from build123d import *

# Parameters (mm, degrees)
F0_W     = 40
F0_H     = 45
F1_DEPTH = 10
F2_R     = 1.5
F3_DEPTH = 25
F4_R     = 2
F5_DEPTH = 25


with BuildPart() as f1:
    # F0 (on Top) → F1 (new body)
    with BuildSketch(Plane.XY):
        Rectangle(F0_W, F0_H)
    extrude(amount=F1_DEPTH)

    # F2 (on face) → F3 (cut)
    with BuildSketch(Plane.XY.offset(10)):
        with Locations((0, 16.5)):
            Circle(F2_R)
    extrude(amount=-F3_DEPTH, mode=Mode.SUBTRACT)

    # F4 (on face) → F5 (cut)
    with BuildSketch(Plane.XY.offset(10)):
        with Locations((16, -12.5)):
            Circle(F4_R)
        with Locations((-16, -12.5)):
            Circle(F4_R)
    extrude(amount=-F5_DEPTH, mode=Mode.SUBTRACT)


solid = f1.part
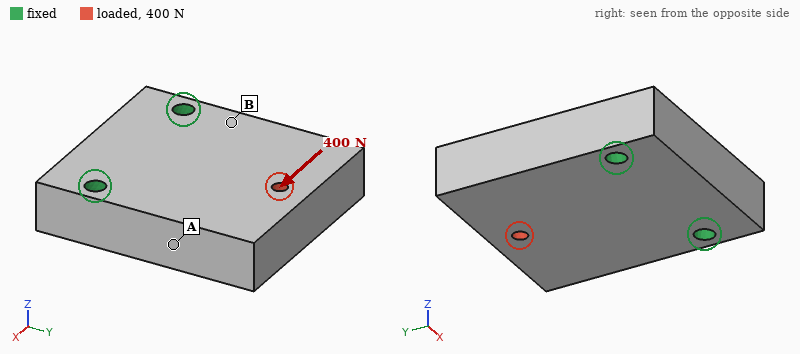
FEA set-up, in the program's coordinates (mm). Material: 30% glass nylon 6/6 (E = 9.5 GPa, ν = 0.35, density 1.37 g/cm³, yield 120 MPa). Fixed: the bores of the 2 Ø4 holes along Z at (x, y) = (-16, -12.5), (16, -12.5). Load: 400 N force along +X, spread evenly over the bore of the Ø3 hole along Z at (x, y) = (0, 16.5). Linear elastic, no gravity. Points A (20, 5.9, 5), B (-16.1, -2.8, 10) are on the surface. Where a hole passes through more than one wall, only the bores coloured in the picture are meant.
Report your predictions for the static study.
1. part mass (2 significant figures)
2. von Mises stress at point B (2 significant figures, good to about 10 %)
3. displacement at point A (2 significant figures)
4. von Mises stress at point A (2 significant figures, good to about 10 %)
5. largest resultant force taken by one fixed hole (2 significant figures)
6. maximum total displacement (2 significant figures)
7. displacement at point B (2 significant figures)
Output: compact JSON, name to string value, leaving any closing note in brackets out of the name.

{"part mass": "24 g", "von Mises stress at point B": "2.7 MPa", "displacement at point A": "11 µm", "von Mises stress at point A": "1.3 MPa", "largest resultant force taken by one fixed hole": "400 N", "maximum total displacement": "19 µm", "displacement at point B": "5.3 µm"}
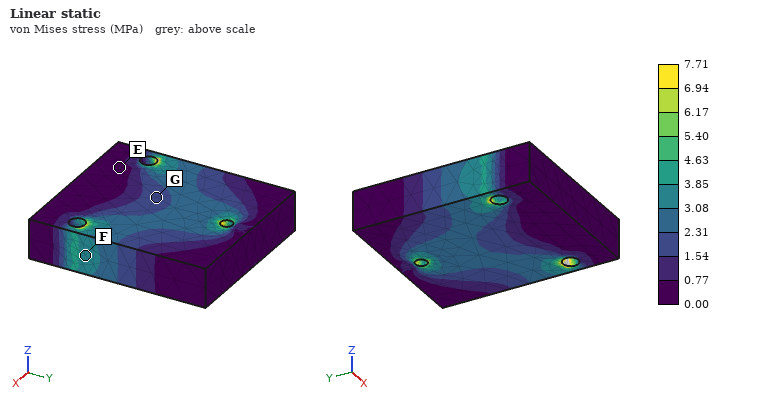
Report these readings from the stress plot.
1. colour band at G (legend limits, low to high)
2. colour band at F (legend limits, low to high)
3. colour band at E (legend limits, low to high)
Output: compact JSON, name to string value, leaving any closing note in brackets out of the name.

{"colour band at G": "1.54 to 2.31 MPa", "colour band at F": "3.08 to 3.85 MPa", "colour band at E": "0.00 to 0.77 MPa"}
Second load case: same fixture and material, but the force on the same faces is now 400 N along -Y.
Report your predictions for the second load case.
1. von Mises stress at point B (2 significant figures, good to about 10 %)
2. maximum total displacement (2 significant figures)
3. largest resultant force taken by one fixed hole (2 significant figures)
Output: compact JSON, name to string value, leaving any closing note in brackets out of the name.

{"von Mises stress at point B": "1.3 MPa", "maximum total displacement": "8.0 µm", "largest resultant force taken by one fixed hole": "200 N"}
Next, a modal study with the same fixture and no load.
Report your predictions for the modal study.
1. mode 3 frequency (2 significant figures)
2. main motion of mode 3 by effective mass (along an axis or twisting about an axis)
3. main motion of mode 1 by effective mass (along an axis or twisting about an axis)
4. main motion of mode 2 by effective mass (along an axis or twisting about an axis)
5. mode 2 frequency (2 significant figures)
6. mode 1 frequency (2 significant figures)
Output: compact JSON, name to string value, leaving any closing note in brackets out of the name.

{"mode 3 frequency": "8200 Hz", "main motion of mode 3 by effective mass": "along X", "main motion of mode 1 by effective mass": "along Z", "main motion of mode 2 by effective mass": "twisting about Y", "mode 2 frequency": "6400 Hz", "mode 1 frequency": "2900 Hz"}
